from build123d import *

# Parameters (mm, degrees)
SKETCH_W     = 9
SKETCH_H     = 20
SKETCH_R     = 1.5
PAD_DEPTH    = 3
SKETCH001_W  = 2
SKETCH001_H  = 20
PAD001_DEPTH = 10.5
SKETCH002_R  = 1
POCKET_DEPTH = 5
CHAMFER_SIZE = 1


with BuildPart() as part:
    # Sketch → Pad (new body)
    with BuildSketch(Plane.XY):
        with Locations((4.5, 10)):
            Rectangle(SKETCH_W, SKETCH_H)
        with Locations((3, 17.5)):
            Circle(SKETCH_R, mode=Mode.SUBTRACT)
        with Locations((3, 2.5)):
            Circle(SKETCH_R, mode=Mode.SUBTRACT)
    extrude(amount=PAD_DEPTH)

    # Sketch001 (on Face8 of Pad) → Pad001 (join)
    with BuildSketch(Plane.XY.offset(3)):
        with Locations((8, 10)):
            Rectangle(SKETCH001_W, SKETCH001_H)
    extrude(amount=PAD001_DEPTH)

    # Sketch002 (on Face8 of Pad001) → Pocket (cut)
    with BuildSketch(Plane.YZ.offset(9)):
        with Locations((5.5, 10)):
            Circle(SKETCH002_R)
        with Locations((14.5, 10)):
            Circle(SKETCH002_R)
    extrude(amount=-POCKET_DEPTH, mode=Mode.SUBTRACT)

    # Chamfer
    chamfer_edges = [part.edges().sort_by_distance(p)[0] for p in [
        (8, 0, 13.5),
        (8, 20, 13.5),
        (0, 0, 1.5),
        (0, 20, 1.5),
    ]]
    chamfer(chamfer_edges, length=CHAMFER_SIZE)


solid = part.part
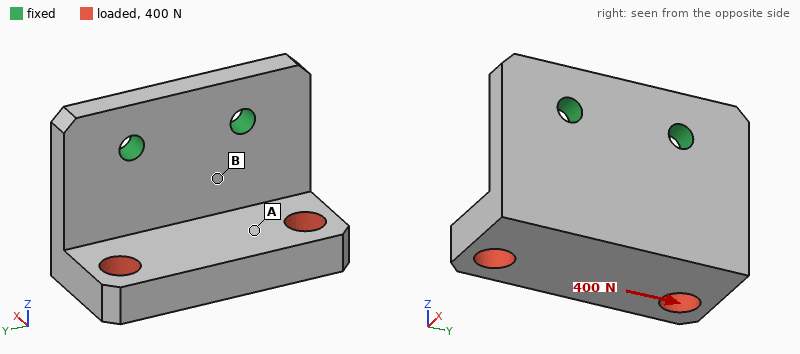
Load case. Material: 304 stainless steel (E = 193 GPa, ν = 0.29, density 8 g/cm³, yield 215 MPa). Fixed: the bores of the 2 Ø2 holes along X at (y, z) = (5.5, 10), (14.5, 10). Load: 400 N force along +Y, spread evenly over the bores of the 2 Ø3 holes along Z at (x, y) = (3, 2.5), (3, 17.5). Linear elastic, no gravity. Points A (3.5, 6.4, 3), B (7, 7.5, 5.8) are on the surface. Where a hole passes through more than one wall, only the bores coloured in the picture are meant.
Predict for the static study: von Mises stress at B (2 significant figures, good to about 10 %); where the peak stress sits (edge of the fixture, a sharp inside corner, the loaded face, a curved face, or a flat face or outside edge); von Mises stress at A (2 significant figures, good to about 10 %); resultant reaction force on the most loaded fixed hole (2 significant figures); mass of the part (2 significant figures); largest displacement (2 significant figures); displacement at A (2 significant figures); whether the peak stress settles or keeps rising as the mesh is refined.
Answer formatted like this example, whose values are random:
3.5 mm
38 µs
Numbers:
85 MPa
edge of the fixture
33 MPa
400 N
7.2 g
20 µm
11 µm
keeps rising
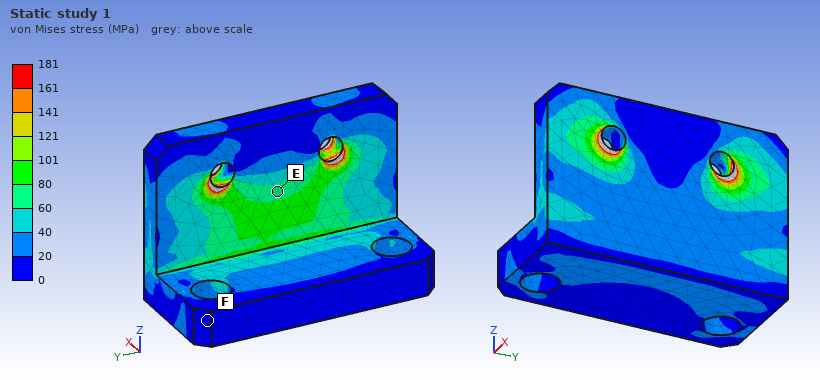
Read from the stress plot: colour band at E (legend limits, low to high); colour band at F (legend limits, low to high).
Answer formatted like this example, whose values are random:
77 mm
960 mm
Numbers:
60 to 80 MPa
0 to 20 MPa
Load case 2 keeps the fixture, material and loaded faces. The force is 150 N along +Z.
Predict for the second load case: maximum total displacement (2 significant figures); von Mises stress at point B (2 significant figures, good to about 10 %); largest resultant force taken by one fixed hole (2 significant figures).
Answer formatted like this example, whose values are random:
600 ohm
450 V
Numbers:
24 µm
54 MPa
75 N
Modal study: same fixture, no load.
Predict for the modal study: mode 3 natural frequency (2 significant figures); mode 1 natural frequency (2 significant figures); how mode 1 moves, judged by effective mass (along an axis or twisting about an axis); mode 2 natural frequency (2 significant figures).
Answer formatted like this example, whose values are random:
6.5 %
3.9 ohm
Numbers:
23 kHz
6800 Hz
along X
12 kHz
